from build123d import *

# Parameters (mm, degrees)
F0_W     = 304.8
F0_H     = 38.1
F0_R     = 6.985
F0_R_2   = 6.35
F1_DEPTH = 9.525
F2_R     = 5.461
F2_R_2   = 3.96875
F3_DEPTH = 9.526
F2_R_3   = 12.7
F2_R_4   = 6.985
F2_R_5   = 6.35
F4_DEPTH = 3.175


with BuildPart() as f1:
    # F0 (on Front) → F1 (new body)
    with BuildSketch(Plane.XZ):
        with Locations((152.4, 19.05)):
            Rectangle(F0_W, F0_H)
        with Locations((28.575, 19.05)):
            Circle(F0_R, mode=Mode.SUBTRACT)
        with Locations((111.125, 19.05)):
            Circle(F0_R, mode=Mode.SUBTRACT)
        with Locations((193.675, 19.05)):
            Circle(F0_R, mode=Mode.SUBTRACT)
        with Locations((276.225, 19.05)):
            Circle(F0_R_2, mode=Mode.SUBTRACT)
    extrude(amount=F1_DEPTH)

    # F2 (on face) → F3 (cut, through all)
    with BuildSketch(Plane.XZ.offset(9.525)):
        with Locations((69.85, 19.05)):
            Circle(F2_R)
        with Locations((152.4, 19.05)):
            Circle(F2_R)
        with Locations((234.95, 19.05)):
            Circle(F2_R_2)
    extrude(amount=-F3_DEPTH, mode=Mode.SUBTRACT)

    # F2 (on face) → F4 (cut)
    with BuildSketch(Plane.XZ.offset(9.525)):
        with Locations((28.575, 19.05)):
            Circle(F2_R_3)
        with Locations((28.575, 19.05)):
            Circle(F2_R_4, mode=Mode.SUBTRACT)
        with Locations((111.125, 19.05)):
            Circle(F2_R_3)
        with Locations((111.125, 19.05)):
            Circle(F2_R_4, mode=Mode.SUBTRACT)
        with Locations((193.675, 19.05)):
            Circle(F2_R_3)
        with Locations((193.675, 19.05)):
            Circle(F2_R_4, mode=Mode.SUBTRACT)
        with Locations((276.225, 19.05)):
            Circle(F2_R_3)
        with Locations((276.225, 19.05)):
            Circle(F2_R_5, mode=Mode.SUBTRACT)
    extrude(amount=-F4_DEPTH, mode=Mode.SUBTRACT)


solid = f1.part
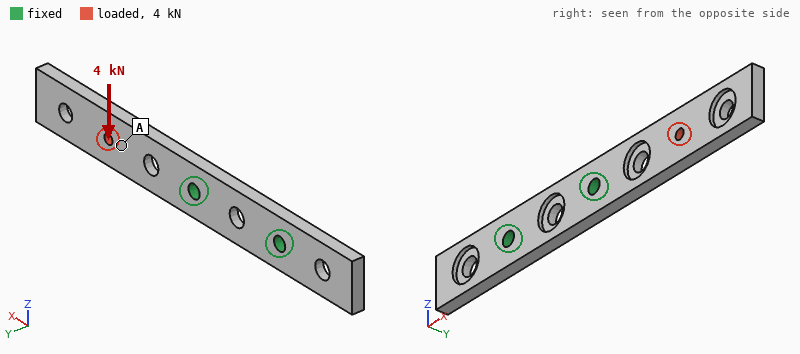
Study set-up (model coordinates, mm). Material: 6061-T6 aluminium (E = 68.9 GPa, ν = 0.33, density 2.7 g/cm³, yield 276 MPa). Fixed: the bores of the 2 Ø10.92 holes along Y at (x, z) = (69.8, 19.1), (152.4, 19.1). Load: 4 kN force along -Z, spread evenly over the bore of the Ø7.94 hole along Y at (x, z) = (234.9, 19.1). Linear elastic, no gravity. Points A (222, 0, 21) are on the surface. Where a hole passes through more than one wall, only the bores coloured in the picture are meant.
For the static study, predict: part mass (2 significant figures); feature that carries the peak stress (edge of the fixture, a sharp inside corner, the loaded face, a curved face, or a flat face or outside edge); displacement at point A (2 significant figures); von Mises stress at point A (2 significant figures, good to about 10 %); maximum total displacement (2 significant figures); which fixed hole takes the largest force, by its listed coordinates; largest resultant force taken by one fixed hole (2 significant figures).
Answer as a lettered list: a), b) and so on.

a) 270 g
b) edge of the fixture
c) 0.36 mm
d) 31 MPa
e) 0.91 mm
f) (152.4, 19.1)
g) 5.9 kN
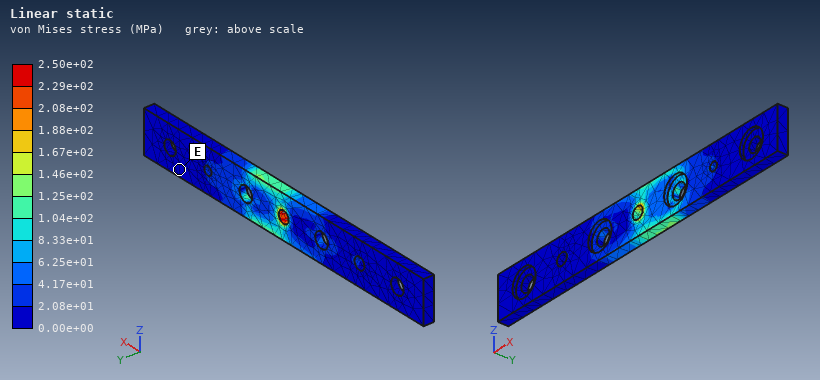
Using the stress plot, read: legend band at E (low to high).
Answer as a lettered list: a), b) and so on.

a) 0.00e+00 to 2.08e+01 MPa
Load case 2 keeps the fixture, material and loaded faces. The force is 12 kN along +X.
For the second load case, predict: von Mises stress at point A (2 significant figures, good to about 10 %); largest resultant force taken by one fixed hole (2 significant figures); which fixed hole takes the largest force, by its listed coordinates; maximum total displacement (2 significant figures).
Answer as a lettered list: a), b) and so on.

a) 37 MPa
b) 11 kN
c) (152.4, 19.1)
d) 0.24 mm
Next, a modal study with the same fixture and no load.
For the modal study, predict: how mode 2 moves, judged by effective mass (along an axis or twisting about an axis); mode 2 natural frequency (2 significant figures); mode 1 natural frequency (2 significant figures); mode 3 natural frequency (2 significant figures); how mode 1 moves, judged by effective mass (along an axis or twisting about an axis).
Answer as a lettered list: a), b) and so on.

a) along Z
b) 1100 Hz
c) 320 Hz
d) 1700 Hz
e) along Y
